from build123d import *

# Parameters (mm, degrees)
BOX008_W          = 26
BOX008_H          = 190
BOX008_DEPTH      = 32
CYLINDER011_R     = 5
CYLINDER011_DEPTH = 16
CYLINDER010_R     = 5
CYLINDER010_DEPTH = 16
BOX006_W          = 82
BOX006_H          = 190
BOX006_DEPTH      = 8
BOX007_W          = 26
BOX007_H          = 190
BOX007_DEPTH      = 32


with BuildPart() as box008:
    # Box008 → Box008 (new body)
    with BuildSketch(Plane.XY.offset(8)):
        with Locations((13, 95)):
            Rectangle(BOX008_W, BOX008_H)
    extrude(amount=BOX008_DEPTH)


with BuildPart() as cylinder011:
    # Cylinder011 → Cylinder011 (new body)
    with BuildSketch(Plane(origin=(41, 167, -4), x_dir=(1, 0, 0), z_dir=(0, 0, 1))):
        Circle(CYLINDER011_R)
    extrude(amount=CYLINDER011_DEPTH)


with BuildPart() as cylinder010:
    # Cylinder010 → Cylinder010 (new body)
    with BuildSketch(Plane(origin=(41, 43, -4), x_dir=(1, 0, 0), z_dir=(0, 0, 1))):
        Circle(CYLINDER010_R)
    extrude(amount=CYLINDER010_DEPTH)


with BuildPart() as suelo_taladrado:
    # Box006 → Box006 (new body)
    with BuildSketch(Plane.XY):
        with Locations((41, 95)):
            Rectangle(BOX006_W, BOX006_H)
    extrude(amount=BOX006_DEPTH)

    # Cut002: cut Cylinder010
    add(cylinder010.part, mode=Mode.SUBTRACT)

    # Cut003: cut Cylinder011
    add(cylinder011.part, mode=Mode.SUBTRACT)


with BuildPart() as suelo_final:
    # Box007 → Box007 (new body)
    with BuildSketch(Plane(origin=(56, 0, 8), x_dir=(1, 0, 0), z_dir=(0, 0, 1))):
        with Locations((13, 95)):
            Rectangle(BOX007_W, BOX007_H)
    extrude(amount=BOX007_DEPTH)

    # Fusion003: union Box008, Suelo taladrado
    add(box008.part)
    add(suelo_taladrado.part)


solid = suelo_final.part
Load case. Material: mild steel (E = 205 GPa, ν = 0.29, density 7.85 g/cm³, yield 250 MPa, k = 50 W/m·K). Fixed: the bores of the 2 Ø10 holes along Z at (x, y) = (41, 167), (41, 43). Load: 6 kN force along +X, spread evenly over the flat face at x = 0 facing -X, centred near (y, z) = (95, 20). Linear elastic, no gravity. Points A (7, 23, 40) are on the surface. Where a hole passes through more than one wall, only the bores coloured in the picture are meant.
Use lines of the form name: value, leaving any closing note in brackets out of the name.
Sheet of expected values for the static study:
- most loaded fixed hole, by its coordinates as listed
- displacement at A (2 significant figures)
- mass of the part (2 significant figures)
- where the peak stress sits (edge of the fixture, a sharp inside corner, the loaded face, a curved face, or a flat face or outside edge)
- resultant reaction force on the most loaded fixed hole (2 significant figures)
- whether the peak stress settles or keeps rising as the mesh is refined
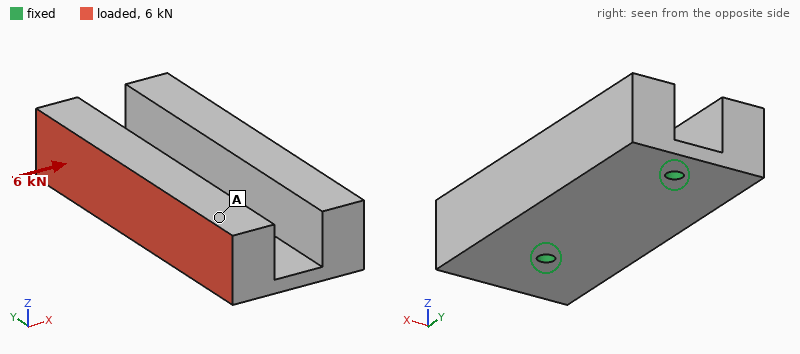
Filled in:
most loaded fixed hole, by its coordinates as listed: (41, 43)
displacement at A: 60 µm
mass of the part: 3.5 kg
where the peak stress sits: edge of the fixture
resultant reaction force on the most loaded fixed hole: 3.5 kN
whether the peak stress settles or keeps rising as the mesh is refined: keeps rising
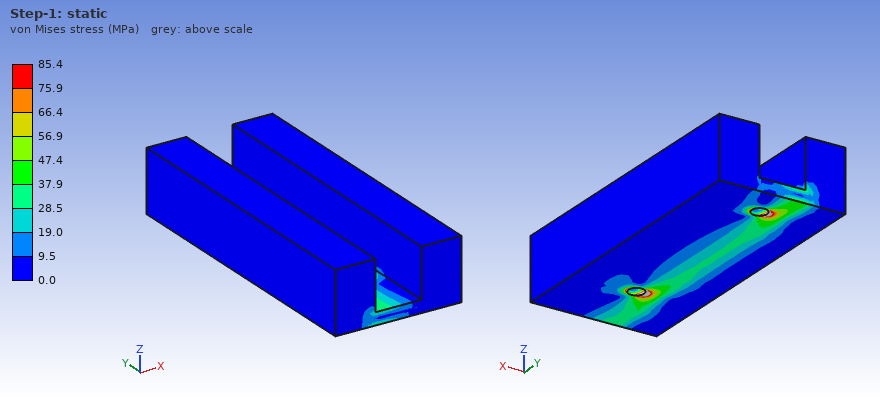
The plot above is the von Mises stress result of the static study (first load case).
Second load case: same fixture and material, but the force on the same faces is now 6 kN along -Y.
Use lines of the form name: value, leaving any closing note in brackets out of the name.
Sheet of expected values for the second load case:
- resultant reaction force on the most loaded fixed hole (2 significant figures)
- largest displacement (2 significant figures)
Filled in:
resultant reaction force on the most loaded fixed hole: 3.8 kN
largest displacement: 5.9 µm
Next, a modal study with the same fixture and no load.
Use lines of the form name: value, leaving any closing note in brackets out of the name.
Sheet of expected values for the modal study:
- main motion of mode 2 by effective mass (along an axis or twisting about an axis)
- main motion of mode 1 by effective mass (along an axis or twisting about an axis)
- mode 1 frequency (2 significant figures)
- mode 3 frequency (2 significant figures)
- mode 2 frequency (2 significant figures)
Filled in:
main motion of mode 2 by effective mass: along Z
main motion of mode 1 by effective mass: along X
mode 1 frequency: 1000 Hz
mode 3 frequency: 2900 Hz
mode 2 frequency: 1400 Hz
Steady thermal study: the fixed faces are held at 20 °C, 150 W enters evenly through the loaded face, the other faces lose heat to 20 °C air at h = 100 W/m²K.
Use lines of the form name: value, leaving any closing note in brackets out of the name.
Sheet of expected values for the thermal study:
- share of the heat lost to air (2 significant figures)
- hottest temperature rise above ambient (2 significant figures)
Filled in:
share of the heat lost to air: 65 %
hottest temperature rise above ambient: 45 K
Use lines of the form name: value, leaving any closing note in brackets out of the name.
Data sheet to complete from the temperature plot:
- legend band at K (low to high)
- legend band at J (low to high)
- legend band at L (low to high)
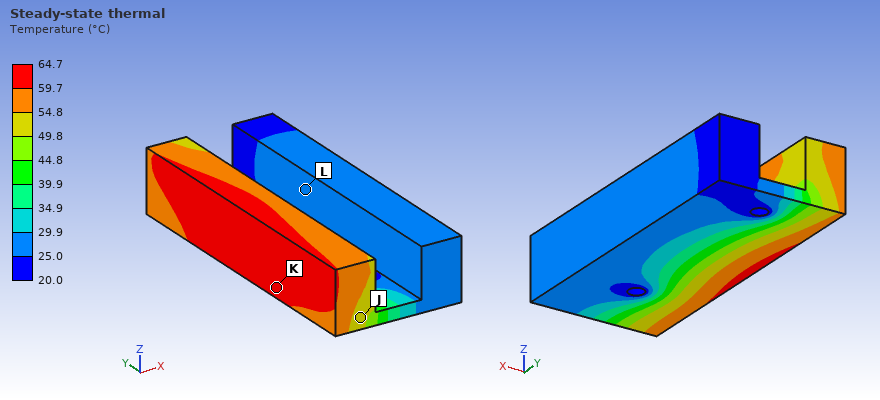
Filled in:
legend band at K: 59.7 to 64.7 °C
legend band at J: 49.8 to 54.8 °C
legend band at L: 25.0 to 29.9 °C
